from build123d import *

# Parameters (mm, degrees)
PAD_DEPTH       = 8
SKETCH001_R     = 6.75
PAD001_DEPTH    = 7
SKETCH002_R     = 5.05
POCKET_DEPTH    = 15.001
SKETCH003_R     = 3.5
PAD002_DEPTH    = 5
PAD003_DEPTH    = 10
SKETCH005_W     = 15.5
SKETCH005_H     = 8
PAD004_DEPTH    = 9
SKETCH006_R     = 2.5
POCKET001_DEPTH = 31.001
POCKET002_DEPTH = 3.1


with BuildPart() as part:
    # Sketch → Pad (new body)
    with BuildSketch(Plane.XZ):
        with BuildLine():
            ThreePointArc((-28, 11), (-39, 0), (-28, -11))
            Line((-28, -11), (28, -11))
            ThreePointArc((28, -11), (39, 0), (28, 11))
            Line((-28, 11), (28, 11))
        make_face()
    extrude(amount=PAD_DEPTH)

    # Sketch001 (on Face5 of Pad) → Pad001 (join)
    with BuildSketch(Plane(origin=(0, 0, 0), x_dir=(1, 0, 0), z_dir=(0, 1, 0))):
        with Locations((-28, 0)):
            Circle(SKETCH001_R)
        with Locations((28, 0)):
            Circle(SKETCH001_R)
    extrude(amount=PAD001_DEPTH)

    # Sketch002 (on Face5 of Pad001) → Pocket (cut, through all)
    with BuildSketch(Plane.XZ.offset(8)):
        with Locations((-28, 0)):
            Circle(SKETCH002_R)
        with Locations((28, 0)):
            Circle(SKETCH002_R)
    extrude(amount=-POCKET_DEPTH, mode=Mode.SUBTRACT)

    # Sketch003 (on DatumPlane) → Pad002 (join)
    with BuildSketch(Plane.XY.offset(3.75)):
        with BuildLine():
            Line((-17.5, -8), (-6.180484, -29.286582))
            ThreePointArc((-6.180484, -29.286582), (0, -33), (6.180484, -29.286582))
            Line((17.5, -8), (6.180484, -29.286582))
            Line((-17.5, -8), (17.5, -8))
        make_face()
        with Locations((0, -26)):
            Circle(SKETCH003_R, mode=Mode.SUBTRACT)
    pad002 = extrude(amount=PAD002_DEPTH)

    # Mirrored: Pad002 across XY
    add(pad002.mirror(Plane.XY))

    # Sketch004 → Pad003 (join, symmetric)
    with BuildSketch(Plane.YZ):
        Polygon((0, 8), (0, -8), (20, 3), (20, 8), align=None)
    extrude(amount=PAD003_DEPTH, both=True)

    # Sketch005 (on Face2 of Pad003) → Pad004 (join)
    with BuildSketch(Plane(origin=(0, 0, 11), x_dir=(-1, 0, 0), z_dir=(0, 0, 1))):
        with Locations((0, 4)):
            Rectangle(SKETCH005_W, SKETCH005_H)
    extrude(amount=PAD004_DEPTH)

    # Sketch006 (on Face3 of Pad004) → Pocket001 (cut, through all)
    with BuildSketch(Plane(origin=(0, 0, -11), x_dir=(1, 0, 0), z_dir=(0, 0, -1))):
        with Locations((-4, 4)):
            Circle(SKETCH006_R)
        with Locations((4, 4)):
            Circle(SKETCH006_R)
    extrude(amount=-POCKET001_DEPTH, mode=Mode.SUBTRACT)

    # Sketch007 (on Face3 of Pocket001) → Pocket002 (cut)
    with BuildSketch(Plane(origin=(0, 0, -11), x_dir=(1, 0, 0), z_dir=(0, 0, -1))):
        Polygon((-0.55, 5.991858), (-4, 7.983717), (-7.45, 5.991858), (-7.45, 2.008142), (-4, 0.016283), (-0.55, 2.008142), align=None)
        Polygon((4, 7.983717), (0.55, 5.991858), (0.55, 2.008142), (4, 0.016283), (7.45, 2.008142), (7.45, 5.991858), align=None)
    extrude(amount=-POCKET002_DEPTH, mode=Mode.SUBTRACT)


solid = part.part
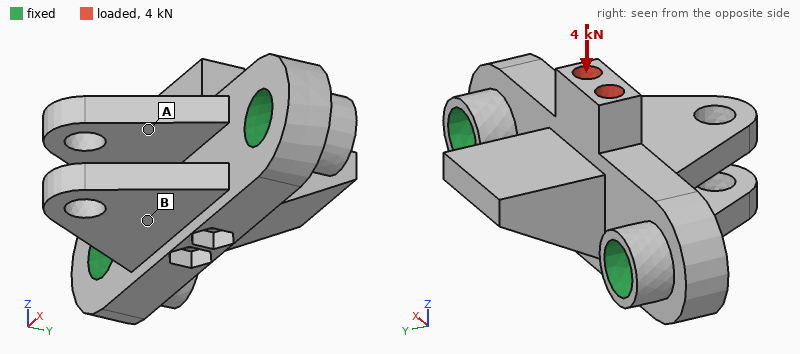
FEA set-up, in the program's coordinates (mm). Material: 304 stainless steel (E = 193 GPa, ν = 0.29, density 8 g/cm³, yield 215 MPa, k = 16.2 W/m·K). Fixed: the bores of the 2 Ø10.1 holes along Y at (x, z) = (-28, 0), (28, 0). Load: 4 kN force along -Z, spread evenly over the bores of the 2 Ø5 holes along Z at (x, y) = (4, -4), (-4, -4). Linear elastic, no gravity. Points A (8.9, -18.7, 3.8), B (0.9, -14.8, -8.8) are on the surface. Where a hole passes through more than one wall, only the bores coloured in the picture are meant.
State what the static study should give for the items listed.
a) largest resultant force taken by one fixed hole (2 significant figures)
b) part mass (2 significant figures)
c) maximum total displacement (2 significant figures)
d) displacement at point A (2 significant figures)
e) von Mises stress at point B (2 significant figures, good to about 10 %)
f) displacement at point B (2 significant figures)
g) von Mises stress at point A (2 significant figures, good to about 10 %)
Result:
2.0 kN
170 g
7.4 µm
5.7 µm
15 MPa
5.9 µm
7.7 MPa
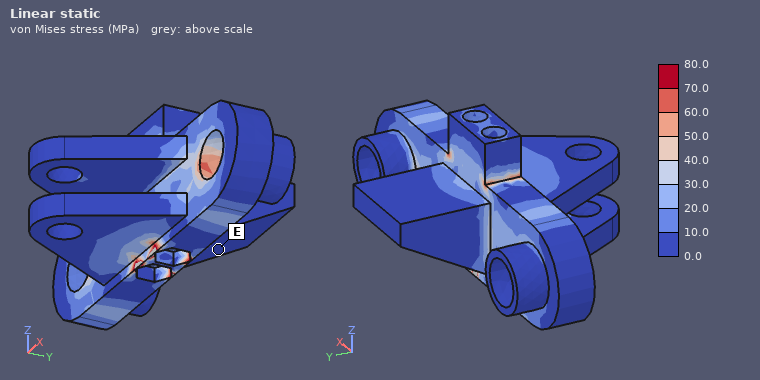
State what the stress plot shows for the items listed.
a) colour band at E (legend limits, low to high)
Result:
0.0 to 10.0 MPa
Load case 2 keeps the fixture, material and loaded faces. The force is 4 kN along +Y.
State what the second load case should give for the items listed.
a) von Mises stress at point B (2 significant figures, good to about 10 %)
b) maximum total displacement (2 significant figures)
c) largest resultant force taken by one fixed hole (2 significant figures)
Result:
11 MPa
25 µm
2.1 kN
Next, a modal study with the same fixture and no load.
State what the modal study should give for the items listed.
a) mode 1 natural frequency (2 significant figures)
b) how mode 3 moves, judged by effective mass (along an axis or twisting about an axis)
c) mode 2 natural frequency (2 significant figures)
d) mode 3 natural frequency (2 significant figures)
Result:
6300 Hz
along Z
8000 Hz
10 kHz
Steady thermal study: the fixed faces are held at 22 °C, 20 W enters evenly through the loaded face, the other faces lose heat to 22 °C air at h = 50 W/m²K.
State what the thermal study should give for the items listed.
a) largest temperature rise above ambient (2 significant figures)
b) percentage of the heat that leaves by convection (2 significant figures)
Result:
70 K
47 %
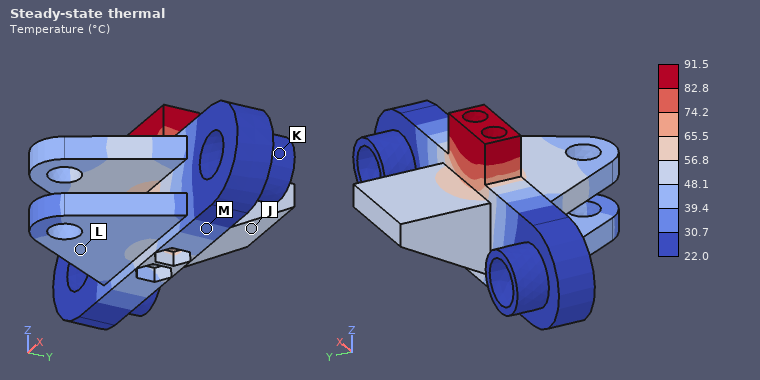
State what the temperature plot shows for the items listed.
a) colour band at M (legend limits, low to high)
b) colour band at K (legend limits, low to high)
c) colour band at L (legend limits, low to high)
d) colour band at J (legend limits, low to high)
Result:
30.7 to 39.4 °C
22.0 to 30.7 °C
39.4 to 48.1 °C
48.1 to 56.8 °C
